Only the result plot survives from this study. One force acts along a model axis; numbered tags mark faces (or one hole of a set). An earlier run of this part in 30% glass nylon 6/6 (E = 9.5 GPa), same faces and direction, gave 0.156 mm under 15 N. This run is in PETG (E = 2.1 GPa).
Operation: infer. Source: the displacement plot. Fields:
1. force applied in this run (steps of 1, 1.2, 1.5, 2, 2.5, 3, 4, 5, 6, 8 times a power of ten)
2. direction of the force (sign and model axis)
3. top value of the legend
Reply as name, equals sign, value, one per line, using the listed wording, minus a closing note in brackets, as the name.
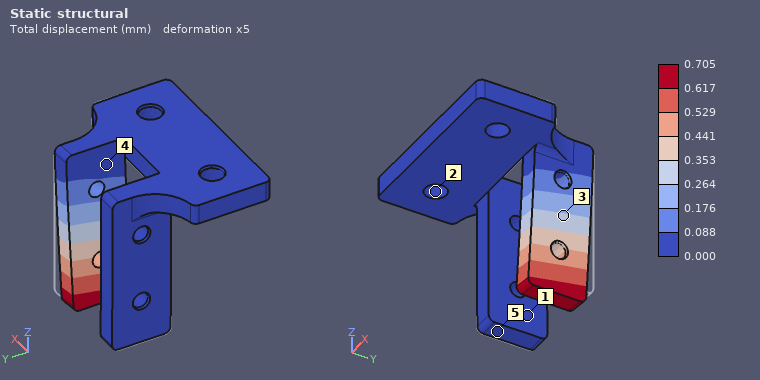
force applied in this run = 15 N
direction of the force = -X
top value of the legend = 0.705 mm
